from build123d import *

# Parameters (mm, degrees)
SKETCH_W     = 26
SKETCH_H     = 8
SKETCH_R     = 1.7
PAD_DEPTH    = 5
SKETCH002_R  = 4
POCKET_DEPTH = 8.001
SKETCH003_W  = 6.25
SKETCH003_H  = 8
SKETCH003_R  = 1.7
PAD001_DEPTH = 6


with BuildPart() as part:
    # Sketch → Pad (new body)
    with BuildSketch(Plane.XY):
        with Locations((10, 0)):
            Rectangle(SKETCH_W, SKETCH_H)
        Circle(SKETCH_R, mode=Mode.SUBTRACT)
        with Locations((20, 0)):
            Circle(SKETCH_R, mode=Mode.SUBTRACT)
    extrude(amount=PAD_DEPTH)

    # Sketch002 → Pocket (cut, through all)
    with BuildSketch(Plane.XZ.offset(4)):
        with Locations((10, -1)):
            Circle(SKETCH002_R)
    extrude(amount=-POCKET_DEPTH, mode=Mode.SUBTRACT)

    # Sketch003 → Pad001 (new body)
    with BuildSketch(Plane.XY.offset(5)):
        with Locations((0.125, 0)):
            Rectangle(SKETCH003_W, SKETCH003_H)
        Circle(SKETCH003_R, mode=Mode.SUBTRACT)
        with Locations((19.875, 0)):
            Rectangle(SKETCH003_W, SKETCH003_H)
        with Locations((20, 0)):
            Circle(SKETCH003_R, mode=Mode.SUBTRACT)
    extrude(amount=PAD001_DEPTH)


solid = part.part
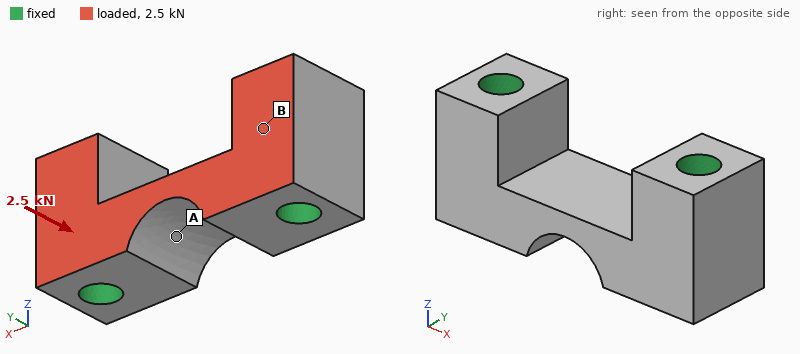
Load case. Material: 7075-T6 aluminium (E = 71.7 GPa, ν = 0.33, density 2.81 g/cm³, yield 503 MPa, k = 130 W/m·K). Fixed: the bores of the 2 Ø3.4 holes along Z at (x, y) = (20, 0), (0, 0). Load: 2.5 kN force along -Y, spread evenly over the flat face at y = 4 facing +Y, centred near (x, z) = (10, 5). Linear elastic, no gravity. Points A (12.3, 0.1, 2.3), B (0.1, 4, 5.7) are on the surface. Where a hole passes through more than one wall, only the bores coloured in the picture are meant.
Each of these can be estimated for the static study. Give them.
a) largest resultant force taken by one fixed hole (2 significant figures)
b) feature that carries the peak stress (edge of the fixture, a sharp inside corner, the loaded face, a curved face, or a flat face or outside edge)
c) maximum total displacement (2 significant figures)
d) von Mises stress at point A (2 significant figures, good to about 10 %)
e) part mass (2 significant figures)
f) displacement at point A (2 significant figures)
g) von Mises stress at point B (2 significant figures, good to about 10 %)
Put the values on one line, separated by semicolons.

1.3 kN; edge of the fixture; 5.1 µm; 6.7 MPa; 3.7 g; 3.5 µm; 22 MPa
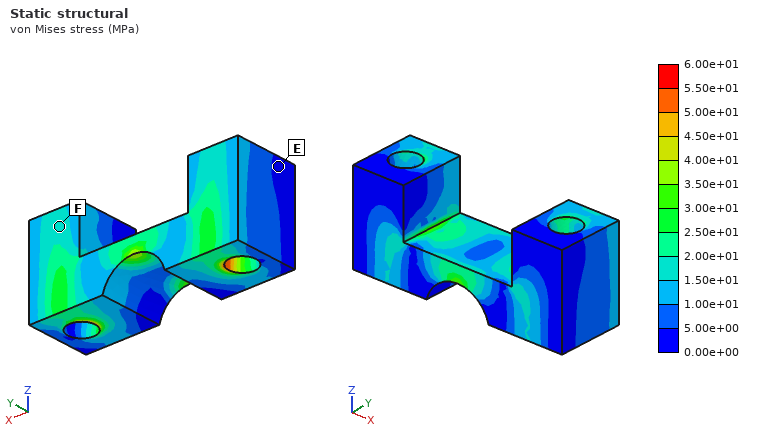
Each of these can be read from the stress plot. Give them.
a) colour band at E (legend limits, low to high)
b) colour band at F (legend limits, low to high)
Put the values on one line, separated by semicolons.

0.00e+00 to 5.00e+00 MPa; 1.50e+01 to 2.00e+01 MPa
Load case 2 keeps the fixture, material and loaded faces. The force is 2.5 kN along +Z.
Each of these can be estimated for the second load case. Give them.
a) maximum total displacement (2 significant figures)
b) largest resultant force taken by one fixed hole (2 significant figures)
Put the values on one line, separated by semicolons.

13 µm; 1.3 kN
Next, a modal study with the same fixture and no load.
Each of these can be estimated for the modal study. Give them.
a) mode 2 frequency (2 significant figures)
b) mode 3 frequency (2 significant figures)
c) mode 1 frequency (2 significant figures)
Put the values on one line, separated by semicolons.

70 kHz; 100 kHz; 68 kHz
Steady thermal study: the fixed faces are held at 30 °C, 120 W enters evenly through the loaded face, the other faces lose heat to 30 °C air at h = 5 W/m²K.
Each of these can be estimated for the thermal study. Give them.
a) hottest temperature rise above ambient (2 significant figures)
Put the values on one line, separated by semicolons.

33 K
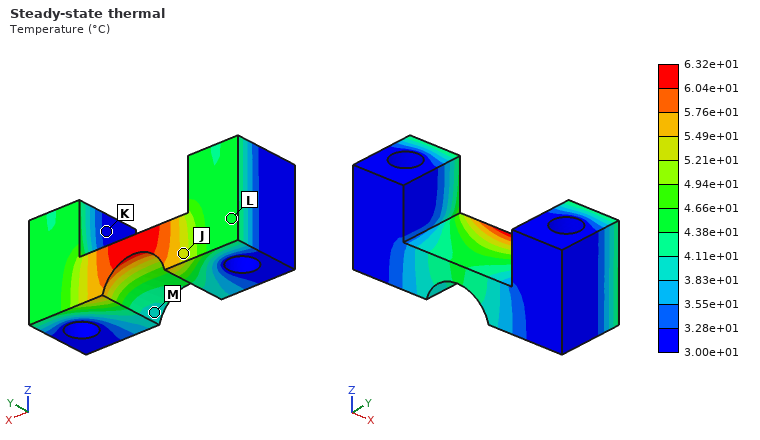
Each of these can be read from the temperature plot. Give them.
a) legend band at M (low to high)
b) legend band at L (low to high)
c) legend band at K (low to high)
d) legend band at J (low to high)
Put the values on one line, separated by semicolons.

3.83e+01 to 4.11e+01 °C; 4.38e+01 to 4.66e+01 °C; 3.00e+01 to 3.28e+01 °C; 5.21e+01 to 5.49e+01 °C
